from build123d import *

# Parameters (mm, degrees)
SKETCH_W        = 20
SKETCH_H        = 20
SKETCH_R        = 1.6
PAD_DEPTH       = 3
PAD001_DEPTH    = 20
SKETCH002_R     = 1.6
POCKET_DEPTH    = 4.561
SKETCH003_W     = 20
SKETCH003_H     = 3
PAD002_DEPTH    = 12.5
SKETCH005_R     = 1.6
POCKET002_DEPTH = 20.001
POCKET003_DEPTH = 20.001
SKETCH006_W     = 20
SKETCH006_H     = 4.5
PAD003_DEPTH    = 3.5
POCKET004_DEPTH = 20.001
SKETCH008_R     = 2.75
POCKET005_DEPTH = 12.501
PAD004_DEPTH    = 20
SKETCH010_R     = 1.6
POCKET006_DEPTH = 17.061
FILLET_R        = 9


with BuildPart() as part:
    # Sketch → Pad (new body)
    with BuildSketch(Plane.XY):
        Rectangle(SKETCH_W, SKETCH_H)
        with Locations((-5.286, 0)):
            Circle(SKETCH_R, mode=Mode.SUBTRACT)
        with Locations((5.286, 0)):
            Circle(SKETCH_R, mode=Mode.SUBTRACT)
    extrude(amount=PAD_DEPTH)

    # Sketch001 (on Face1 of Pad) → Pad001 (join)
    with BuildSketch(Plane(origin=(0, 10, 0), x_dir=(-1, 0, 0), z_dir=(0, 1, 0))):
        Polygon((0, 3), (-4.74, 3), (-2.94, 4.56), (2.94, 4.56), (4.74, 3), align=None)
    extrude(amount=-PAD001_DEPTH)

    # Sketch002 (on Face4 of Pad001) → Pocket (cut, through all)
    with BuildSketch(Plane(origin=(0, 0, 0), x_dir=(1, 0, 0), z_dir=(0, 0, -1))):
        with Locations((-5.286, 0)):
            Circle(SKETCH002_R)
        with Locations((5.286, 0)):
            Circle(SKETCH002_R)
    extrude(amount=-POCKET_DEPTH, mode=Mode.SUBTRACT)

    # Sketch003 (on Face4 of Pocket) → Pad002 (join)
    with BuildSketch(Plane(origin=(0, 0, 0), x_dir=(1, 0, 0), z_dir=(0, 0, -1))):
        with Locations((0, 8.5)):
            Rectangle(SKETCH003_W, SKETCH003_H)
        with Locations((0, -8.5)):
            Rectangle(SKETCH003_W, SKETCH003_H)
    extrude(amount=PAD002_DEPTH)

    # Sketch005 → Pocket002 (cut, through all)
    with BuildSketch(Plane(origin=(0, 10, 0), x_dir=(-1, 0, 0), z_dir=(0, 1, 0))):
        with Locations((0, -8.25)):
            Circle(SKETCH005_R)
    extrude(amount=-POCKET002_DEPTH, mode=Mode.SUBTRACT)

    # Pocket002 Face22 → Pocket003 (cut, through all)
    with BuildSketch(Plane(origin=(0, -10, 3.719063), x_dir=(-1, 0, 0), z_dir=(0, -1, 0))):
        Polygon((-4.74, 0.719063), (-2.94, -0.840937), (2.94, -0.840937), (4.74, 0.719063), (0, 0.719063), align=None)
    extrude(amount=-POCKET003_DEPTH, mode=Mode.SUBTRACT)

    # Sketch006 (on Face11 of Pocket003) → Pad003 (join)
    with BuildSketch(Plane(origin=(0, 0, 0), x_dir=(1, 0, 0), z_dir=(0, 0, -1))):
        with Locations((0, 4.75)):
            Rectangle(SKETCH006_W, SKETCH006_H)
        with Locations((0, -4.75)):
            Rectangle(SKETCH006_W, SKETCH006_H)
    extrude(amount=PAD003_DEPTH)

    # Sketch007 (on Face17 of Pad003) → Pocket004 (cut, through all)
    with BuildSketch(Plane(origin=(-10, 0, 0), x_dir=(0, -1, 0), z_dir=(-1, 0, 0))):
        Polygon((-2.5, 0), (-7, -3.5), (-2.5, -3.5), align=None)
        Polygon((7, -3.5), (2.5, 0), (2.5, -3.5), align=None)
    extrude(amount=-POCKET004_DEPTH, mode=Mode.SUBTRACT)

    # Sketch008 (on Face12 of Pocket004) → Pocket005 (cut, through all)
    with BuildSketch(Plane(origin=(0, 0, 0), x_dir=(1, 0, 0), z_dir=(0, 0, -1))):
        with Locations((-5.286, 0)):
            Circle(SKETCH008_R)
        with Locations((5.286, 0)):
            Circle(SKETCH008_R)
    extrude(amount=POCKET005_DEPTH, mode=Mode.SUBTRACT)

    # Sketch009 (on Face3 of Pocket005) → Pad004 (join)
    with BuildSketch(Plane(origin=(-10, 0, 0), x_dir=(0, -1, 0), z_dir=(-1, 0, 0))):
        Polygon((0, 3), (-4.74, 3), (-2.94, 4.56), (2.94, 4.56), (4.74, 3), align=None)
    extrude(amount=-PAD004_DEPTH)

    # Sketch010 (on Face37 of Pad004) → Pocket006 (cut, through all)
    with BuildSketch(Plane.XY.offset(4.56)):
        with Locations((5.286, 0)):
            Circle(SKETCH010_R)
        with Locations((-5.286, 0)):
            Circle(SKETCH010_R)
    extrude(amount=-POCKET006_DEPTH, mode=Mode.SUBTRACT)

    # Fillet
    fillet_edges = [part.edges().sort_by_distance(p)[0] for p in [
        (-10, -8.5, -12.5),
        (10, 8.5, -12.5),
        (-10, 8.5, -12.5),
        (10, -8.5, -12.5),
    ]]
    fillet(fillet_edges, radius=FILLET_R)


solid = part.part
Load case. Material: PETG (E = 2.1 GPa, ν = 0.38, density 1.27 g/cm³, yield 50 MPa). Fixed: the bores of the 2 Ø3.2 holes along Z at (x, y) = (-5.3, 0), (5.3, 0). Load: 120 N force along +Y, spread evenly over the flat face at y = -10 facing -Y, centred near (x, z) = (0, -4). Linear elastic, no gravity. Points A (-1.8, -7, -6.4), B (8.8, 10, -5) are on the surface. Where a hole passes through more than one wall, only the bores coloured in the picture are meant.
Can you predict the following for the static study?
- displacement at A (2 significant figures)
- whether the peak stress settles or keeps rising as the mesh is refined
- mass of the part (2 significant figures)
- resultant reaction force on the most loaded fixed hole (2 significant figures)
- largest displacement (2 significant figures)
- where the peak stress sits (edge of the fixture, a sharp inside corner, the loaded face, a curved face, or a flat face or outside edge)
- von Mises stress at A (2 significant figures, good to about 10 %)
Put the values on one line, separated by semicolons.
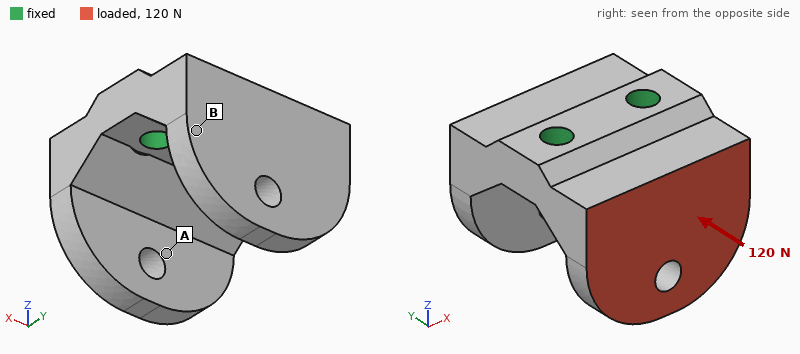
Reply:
0.16 mm; keeps rising; 3.7 g; 61 N; 0.34 mm; edge of the fixture; 4.8 MPa
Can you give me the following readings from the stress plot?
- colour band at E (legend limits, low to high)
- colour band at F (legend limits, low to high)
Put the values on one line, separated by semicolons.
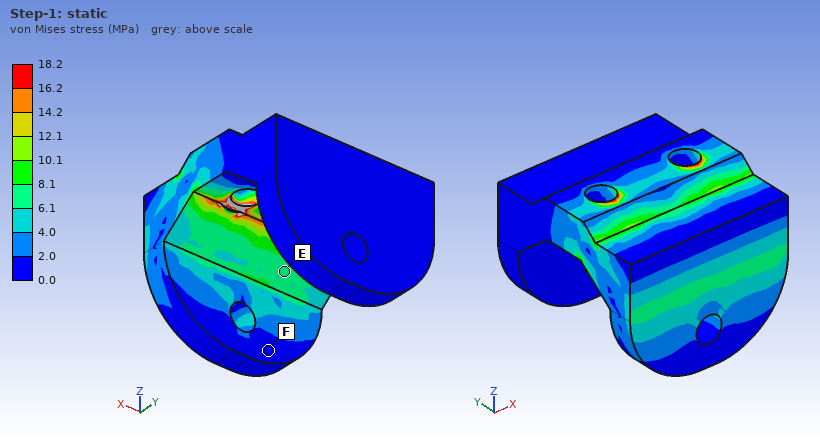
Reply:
6.1 to 8.1 MPa; 0.0 to 2.0 MPa
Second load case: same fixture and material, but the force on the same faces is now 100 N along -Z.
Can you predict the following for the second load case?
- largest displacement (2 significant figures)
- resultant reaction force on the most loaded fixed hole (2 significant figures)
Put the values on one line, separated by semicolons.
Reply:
0.29 mm; 50 N
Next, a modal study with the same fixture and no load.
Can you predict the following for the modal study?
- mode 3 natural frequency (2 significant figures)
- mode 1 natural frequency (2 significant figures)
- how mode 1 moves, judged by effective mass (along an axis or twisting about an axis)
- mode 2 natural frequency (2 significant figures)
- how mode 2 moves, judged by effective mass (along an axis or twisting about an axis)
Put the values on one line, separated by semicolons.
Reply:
5600 Hz; 3300 Hz; along Y; 3500 Hz; along Z
